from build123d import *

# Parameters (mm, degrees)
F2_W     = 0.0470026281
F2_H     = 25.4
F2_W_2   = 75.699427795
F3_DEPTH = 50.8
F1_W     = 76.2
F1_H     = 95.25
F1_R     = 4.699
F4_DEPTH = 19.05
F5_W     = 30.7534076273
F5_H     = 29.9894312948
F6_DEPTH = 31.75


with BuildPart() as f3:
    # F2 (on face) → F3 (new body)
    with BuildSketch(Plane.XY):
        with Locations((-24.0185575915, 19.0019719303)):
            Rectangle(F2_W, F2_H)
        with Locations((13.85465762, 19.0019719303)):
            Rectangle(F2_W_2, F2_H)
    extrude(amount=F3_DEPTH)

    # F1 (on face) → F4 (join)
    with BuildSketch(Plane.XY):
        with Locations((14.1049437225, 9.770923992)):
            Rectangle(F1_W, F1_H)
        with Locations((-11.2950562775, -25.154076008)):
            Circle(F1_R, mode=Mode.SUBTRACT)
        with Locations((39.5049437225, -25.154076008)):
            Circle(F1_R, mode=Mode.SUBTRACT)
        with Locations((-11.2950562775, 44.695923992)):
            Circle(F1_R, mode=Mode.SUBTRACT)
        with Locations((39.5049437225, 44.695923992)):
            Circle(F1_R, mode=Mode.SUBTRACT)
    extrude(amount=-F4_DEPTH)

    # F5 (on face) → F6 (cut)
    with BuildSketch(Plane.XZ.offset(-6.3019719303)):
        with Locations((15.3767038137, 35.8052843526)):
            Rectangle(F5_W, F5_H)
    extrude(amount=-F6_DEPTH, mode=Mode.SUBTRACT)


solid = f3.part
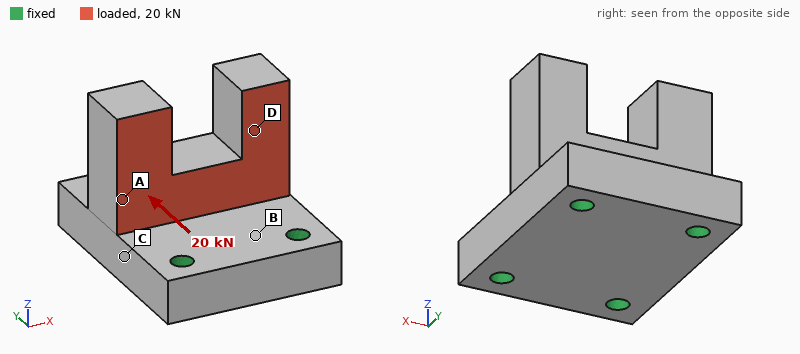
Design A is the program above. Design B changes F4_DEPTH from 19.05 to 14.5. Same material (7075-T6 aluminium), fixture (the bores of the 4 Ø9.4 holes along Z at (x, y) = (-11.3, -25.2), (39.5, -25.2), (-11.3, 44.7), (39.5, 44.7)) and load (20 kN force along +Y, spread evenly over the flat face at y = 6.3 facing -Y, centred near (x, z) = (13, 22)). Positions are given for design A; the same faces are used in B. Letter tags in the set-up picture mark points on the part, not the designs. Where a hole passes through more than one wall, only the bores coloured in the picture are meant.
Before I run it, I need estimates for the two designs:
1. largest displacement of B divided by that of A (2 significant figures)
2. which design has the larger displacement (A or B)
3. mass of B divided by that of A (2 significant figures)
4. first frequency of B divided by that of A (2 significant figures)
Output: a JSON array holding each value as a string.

["1.2", "B", "0.85", "0.89"]
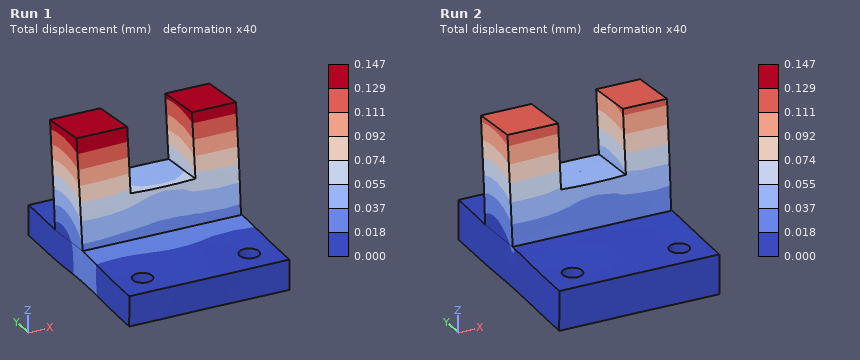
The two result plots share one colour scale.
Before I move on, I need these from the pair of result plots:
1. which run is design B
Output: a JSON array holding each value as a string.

["Run 1"]
